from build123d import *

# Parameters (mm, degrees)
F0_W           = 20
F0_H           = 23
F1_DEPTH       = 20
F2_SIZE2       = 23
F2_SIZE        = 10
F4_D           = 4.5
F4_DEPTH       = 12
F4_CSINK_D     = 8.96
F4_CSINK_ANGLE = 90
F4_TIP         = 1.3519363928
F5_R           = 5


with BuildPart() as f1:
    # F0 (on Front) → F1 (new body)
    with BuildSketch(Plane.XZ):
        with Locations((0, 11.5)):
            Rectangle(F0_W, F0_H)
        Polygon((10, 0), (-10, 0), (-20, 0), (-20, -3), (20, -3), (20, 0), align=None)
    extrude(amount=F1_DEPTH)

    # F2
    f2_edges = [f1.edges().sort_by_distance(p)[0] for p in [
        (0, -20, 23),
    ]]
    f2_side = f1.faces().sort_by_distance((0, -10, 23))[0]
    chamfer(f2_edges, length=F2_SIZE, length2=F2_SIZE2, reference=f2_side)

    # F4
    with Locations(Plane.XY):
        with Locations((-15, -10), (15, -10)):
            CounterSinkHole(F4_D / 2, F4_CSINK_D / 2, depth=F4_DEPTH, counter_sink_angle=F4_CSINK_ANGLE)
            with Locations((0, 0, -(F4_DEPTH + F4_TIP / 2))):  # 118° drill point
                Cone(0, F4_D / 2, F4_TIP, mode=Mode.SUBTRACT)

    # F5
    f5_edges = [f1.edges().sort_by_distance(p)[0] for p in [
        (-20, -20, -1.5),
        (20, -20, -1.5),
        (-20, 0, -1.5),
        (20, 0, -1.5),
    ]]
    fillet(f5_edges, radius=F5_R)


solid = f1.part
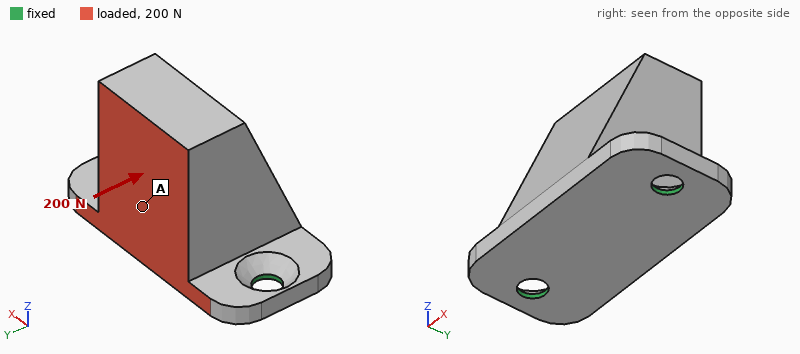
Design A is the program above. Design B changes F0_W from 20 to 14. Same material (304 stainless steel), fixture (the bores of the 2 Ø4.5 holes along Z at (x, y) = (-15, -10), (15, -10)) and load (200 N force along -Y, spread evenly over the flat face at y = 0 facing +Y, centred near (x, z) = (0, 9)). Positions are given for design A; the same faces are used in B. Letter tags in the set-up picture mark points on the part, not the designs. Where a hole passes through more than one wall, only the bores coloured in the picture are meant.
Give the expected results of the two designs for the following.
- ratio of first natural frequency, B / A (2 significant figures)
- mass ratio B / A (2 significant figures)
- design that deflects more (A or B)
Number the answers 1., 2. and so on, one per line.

1. 1.0
2. 0.77
3. B
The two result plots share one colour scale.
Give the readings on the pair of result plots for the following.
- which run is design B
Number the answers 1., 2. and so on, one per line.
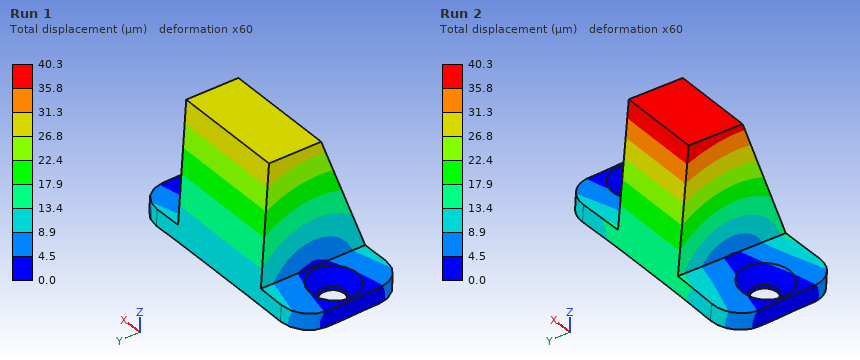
1. Run 2
